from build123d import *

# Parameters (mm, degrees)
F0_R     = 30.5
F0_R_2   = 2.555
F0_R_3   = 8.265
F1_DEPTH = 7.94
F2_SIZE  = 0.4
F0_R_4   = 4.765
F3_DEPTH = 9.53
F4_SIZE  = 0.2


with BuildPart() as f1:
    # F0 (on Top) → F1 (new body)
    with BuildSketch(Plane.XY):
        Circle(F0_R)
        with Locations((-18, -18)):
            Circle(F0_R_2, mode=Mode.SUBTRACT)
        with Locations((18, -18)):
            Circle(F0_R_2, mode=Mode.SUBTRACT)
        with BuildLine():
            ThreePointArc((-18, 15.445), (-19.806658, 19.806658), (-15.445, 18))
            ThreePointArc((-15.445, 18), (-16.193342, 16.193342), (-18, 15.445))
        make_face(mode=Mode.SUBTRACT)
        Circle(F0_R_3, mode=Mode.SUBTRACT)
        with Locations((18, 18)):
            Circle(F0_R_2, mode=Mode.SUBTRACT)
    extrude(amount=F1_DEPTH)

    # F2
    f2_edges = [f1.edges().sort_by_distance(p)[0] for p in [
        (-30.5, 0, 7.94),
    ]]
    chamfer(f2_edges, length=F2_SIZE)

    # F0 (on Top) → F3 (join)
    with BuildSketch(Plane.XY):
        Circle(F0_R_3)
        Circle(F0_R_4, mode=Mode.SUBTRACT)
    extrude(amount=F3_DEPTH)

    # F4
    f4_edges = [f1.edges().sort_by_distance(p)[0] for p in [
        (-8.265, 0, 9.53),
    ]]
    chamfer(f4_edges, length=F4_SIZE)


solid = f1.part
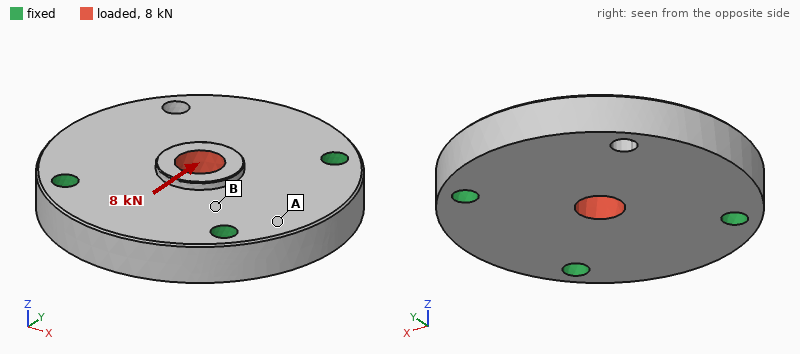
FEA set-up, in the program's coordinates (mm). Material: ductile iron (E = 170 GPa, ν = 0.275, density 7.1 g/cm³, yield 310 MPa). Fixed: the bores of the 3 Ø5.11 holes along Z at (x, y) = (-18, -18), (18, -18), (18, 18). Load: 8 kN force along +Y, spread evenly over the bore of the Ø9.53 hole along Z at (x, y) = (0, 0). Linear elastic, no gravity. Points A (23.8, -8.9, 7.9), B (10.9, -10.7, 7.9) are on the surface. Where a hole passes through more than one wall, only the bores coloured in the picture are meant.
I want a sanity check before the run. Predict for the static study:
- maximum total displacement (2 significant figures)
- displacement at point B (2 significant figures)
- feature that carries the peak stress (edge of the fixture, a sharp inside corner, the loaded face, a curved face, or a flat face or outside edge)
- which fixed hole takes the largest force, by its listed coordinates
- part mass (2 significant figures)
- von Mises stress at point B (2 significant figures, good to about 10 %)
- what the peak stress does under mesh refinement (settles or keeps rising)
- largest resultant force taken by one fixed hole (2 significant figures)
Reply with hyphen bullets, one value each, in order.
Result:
- 5.3 µm
- 1.6 µm
- edge of the fixture
- (-18, -18)
- 160 g
- 28 MPa
- keeps rising
- 3.4 kN
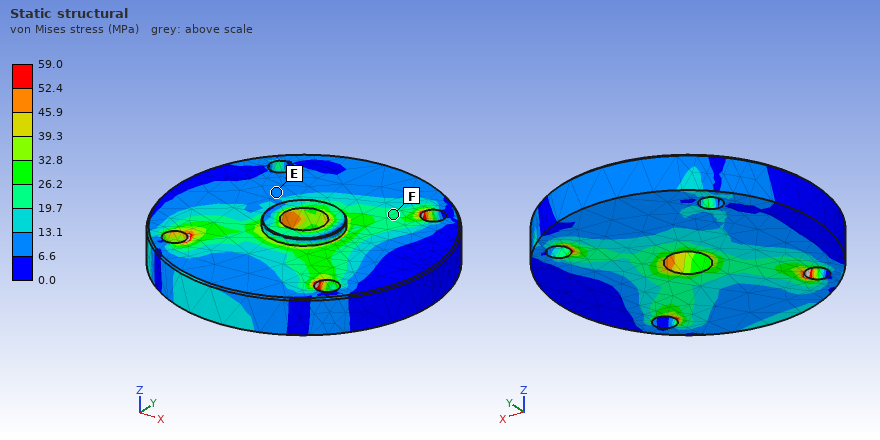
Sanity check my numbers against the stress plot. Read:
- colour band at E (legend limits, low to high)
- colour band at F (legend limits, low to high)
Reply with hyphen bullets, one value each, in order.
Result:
- 6.6 to 13.1 MPa
- 19.7 to 26.2 MPa
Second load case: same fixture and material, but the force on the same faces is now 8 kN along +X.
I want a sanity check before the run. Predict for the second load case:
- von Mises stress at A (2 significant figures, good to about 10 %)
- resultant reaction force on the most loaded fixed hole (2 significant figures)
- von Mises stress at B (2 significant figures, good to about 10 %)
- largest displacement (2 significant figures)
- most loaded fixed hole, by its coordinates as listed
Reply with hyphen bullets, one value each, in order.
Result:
- 10 MPa
- 3.4 kN
- 28 MPa
- 5.3 µm
- (18, 18)
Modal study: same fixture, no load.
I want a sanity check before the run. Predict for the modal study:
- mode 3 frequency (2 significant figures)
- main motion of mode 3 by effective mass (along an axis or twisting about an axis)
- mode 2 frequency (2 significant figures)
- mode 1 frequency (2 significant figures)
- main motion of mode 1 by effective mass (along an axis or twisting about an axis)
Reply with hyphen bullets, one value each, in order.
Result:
- 19 kHz
- along Z
- 16 kHz
- 6300 Hz
- along Z
